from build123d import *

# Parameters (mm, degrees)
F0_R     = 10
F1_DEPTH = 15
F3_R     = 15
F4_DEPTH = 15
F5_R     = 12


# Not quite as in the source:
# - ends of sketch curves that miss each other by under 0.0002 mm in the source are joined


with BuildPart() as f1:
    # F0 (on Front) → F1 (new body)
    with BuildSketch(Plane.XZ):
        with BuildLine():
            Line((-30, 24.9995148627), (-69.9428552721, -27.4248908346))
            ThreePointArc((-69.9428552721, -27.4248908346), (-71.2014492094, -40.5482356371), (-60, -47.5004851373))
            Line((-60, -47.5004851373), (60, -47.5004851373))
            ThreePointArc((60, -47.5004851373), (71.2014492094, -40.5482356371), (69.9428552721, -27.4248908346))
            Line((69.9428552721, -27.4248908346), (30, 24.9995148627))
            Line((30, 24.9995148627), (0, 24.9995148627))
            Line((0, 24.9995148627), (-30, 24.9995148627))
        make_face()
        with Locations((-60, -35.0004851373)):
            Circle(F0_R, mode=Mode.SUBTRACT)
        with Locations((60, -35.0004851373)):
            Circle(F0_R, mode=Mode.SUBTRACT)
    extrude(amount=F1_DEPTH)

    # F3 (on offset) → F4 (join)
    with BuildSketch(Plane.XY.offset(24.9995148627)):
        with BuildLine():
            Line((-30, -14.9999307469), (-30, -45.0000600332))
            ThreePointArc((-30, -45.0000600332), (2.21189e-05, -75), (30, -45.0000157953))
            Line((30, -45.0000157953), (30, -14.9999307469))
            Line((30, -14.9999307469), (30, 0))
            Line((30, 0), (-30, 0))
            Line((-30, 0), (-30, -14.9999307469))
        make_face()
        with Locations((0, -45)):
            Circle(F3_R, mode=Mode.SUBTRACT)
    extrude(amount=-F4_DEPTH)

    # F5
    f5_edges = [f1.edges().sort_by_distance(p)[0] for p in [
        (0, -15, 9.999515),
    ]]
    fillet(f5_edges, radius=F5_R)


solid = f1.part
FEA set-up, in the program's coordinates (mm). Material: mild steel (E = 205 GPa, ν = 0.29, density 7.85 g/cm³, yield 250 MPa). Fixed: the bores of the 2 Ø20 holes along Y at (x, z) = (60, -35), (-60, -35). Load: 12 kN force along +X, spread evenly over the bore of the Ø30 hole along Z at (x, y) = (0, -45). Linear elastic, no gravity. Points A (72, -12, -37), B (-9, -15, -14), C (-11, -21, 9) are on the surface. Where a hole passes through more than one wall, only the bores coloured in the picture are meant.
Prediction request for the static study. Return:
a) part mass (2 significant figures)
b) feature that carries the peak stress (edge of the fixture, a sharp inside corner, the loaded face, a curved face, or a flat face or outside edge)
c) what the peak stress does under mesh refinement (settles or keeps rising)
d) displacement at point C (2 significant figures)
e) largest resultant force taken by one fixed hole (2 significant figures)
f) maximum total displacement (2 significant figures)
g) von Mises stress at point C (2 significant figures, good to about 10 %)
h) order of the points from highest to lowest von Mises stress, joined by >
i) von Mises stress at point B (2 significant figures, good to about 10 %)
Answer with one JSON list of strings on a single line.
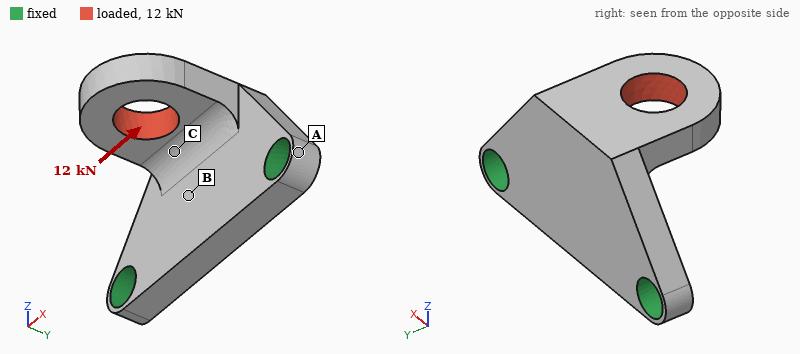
["1.2 kg", "a sharp inside corner", "keeps rising", "0.023 mm", "9.3 kN", "0.11 mm", "83 MPa", "C > B > A", "52 MPa"]
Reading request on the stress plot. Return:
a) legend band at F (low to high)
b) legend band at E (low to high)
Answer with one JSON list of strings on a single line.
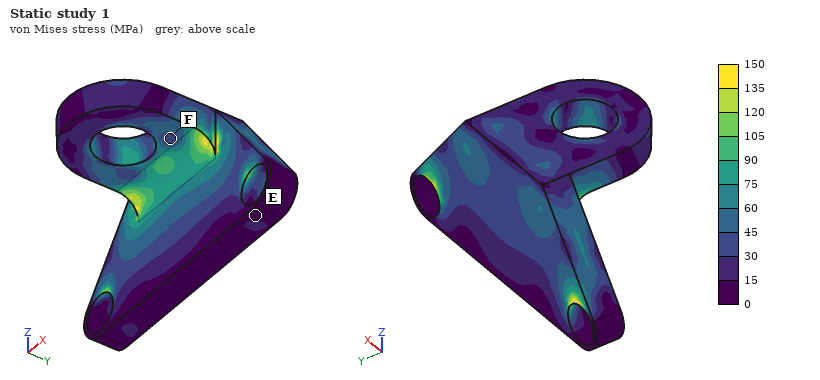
["30 to 45 MPa", "0 to 15 MPa"]
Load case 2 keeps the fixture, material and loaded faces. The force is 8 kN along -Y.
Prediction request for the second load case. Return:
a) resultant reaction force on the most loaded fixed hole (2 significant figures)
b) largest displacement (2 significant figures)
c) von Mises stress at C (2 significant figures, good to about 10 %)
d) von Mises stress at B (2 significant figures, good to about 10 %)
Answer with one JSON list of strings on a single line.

["4.0 kN", "0.19 mm", "24 MPa", "42 MPa"]
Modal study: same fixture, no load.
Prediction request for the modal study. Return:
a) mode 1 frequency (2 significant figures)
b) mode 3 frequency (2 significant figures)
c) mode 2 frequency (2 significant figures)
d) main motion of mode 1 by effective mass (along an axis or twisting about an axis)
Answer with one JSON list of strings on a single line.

["1600 Hz", "3600 Hz", "3500 Hz", "along Y"]
